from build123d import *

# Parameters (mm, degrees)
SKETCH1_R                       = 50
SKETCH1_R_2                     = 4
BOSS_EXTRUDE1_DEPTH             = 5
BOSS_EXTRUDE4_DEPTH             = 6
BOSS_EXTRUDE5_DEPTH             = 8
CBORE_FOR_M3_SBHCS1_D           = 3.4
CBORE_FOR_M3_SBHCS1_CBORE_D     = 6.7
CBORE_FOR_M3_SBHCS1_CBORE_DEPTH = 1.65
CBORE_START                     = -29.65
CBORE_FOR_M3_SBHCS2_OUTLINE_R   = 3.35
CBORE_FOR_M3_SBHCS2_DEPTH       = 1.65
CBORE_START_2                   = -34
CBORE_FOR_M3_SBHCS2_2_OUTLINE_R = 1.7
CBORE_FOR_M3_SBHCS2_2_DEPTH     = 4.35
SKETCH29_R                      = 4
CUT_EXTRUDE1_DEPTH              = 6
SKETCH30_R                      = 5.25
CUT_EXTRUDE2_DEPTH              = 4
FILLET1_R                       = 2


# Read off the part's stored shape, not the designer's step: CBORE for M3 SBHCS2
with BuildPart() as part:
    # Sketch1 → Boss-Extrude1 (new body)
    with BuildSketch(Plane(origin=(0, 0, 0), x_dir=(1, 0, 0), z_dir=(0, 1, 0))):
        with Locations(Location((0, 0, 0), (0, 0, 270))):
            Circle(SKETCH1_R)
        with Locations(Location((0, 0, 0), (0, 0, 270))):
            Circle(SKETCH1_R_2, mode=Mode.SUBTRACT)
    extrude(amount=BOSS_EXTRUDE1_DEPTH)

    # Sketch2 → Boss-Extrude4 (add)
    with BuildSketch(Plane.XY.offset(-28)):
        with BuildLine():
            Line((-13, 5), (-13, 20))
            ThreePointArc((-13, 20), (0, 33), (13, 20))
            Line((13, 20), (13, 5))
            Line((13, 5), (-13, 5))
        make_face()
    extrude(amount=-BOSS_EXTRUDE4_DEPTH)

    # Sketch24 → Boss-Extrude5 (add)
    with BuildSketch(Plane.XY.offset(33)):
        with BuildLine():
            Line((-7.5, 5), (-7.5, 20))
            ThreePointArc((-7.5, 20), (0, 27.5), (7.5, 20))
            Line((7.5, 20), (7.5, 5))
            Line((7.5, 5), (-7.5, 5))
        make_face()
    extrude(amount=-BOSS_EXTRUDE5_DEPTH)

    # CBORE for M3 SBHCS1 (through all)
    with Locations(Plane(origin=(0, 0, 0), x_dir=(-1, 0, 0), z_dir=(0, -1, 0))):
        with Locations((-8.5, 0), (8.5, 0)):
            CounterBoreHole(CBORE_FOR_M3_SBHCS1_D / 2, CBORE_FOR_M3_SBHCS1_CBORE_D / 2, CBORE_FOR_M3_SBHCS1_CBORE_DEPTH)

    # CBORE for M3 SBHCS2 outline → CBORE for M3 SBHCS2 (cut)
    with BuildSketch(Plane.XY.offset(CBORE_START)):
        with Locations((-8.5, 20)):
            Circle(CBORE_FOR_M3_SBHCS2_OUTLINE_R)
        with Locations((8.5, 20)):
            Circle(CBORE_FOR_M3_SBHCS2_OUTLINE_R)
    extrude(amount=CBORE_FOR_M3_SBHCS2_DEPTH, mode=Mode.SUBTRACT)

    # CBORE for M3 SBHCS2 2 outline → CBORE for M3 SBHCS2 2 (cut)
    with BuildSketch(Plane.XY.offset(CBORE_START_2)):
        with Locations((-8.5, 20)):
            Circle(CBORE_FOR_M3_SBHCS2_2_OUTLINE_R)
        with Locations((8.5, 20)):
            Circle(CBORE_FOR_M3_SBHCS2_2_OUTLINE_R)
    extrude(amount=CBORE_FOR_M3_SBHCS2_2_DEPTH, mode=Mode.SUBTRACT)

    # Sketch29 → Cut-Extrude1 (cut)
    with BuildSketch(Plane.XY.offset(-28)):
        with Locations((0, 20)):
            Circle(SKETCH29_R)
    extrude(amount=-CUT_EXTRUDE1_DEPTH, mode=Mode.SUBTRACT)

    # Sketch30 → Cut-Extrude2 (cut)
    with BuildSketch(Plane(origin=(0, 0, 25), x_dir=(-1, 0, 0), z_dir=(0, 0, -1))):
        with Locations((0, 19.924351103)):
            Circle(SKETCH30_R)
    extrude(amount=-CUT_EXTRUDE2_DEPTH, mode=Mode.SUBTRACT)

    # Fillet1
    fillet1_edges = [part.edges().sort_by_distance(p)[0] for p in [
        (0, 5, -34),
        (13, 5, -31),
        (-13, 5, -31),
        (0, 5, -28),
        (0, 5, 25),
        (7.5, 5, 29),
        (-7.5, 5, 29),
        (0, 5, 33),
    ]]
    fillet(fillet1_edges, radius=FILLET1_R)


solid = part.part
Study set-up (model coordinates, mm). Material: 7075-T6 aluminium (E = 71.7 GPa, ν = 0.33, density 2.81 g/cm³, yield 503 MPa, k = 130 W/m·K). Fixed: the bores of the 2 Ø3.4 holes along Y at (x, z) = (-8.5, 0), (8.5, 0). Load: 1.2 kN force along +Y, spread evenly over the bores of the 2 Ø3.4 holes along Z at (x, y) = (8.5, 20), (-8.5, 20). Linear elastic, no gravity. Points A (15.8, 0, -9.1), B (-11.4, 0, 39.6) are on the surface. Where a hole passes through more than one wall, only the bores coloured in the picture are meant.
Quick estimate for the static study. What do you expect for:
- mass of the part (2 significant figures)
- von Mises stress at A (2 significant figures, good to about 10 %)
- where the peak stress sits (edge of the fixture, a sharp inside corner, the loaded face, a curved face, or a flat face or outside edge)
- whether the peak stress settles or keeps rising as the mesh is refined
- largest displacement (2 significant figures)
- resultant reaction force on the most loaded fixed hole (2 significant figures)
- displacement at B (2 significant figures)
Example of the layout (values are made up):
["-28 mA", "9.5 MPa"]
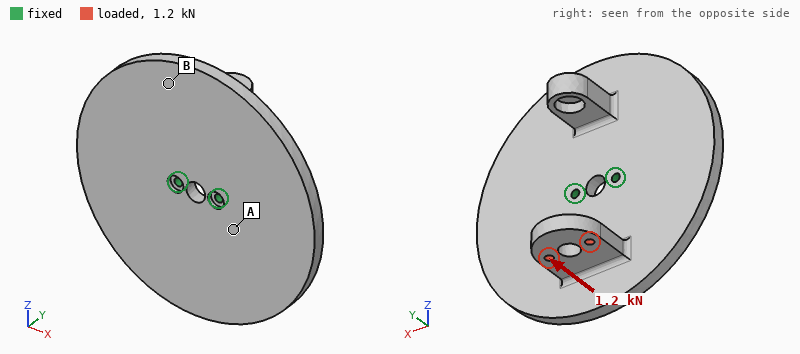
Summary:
["130 g", "88 MPa", "edge of the fixture", "keeps rising", "0.87 mm", "640 N", "0.36 mm"]
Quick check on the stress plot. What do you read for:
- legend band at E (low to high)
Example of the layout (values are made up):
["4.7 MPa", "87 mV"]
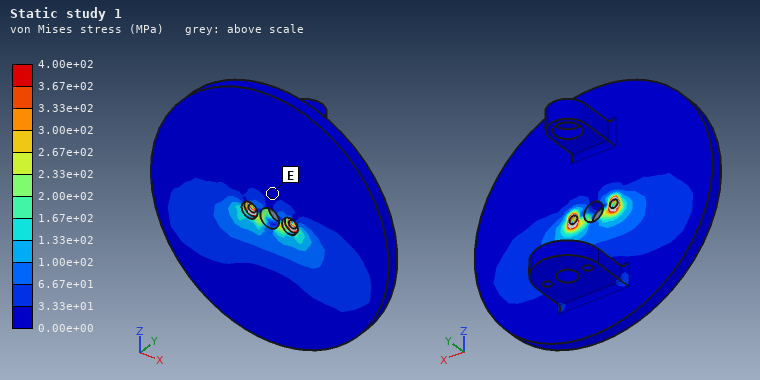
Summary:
["0.00e+00 to 3.33e+01 MPa"]
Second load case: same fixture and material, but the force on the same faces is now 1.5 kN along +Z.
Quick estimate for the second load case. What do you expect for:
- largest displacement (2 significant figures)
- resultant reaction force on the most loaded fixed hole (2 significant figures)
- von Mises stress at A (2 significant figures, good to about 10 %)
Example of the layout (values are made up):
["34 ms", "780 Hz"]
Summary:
["0.89 mm", "750 N", "72 MPa"]
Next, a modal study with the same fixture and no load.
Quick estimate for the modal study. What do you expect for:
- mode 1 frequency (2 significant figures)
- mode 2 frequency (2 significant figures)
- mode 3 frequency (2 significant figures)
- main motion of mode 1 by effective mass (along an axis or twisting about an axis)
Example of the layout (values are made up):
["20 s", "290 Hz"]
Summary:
["920 Hz", "1700 Hz", "1700 Hz", "twisting about X"]
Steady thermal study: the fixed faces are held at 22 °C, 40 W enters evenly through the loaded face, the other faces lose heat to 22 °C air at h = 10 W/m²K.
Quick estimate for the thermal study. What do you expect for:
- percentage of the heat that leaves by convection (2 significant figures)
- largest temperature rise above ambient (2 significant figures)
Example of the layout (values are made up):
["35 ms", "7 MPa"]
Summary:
["10 %", "80 K"]
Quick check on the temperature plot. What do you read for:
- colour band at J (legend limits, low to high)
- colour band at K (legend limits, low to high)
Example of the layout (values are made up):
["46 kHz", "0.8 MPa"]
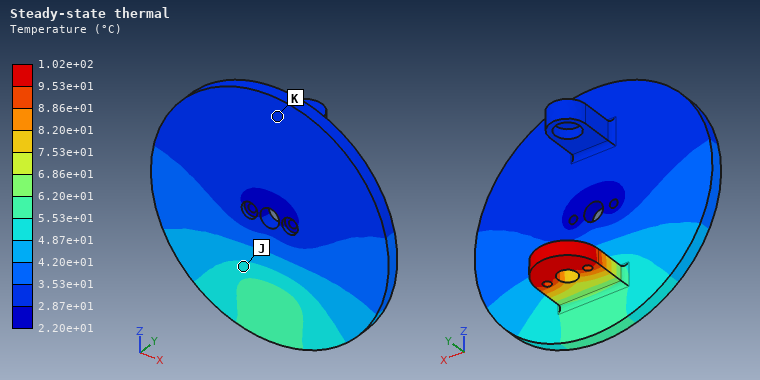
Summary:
["4.87e+01 to 5.53e+01 °C", "2.87e+01 to 3.53e+01 °C"]
